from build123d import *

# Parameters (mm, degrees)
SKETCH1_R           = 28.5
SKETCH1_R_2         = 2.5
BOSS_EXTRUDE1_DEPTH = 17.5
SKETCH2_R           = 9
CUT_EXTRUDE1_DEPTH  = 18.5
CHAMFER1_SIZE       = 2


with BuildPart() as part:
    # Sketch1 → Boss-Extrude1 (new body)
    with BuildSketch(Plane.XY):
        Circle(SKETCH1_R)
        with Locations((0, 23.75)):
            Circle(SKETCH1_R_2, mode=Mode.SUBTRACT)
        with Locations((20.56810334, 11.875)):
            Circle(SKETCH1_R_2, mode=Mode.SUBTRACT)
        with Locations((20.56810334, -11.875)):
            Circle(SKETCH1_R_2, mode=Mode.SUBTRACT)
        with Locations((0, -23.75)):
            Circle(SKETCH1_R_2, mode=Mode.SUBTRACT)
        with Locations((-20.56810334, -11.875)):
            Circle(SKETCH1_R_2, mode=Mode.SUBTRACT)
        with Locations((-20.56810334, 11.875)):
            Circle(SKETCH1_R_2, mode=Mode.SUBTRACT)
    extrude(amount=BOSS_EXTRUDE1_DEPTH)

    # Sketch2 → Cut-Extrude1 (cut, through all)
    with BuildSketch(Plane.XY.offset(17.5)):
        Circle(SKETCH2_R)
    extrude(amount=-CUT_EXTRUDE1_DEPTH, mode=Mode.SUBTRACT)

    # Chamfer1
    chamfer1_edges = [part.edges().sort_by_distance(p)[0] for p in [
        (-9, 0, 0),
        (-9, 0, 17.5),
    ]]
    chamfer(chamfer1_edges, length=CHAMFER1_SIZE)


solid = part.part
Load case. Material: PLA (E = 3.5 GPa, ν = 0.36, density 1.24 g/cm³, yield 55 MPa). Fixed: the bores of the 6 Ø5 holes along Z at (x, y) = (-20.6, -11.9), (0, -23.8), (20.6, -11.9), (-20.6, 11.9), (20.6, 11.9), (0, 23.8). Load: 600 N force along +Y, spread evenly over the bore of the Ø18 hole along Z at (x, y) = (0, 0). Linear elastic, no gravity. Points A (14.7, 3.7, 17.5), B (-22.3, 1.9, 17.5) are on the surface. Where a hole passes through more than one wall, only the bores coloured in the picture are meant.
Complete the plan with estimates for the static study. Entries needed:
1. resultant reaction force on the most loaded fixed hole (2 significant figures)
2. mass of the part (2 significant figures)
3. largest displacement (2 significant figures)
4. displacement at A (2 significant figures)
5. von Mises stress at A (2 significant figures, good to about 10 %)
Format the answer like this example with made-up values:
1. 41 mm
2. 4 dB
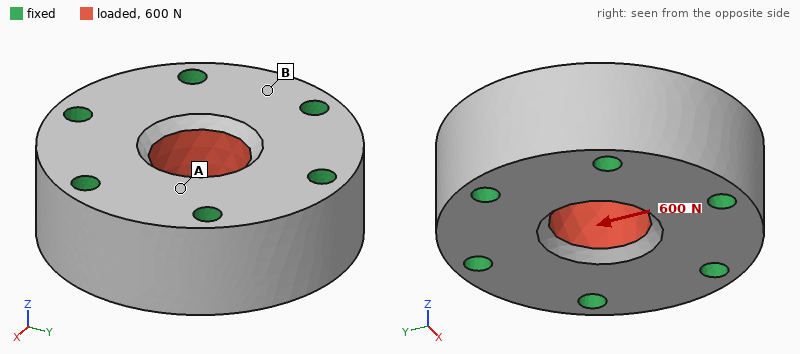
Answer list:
1. 150 N
2. 47 g
3. 3.2 µm
4. 0.93 µm
5. 0.34 MPa
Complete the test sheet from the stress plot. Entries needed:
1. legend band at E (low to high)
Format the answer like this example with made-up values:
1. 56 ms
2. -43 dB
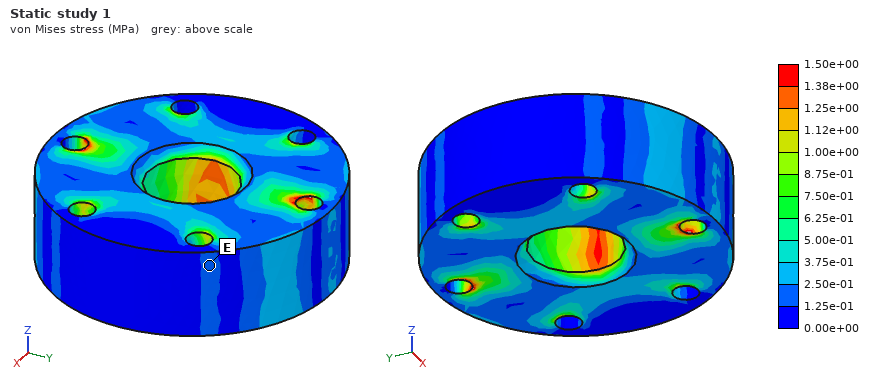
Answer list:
1. 1.25e-01 to 2.50e-01 MPa
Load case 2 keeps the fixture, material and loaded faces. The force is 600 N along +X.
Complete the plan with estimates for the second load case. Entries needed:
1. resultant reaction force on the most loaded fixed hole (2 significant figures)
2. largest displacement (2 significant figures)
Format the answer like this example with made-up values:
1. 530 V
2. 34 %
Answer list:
1. 130 N
2. 3.3 µm
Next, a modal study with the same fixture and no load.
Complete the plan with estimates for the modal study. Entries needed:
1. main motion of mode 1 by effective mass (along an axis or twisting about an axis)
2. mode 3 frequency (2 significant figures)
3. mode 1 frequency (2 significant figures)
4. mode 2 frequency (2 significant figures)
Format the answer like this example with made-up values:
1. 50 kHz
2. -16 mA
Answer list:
1. along Z
2. 17 kHz
3. 14 kHz
4. 17 kHz
